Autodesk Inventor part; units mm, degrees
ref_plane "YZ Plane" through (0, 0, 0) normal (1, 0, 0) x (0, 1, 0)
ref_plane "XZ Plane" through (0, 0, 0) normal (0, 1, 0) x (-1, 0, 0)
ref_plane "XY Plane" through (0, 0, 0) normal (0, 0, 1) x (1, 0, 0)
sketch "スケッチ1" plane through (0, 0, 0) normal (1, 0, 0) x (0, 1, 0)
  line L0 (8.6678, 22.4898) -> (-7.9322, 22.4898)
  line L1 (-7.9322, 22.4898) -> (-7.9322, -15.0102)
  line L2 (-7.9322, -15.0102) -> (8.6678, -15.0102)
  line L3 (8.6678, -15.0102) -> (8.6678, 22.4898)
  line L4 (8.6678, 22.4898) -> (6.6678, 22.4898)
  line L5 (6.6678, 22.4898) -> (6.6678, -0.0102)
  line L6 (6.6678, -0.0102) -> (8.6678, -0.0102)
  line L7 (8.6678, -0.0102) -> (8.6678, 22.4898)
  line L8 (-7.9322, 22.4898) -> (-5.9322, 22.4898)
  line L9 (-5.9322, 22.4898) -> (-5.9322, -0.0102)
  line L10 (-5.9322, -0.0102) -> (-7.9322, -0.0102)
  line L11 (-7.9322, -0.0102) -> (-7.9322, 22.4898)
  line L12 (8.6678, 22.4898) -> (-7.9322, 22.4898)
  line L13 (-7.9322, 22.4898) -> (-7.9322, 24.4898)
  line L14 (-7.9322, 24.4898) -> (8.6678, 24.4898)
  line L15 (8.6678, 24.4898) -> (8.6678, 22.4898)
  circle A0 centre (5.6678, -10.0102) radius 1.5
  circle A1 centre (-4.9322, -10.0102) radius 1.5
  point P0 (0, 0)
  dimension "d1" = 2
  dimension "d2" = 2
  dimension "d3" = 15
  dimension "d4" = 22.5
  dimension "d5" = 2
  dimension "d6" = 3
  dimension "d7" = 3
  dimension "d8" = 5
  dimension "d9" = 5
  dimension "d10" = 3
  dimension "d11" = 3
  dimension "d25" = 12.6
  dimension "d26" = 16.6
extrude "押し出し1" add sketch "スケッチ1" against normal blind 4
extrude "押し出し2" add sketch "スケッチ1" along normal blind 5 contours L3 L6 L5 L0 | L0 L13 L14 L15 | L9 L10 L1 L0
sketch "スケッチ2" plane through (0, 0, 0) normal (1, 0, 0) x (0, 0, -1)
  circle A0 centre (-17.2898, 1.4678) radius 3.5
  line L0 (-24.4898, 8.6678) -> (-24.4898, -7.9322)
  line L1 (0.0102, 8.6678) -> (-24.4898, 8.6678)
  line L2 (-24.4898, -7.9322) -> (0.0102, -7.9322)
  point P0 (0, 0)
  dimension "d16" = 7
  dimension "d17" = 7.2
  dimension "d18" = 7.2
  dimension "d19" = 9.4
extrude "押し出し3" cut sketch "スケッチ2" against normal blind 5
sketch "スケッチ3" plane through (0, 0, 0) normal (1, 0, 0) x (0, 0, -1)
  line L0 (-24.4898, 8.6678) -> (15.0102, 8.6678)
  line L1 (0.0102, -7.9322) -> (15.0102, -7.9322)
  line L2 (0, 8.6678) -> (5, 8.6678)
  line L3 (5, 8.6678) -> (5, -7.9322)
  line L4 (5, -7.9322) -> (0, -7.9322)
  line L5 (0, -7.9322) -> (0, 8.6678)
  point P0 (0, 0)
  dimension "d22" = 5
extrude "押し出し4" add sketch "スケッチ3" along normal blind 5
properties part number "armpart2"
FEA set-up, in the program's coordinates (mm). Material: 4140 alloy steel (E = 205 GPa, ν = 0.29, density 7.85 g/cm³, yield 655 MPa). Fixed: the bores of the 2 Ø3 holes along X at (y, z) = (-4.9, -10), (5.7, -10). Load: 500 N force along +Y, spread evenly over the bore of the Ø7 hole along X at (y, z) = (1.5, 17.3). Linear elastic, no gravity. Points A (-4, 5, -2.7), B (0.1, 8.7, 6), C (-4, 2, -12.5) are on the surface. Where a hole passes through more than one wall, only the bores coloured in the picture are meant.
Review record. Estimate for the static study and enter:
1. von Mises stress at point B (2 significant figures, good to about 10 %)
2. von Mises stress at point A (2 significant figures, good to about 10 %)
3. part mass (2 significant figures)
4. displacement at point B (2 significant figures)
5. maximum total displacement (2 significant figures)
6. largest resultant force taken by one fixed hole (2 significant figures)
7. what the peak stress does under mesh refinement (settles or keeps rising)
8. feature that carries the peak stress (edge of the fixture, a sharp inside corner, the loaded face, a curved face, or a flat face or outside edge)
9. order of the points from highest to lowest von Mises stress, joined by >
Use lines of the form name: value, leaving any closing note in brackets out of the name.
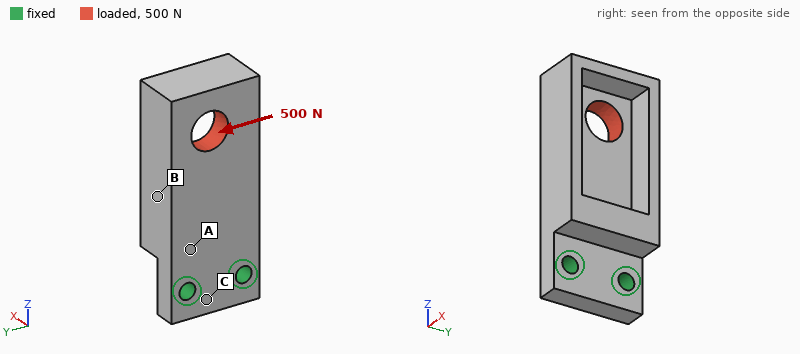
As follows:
von Mises stress at point B: 19 MPa
von Mises stress at point A: 37 MPa
part mass: 27 g
displacement at point B: 6.5 µm
maximum total displacement: 18 µm
largest resultant force taken by one fixed hole: 1.2 kN
what the peak stress does under mesh refinement: keeps rising
feature that carries the peak stress: edge of the fixture
order of the points from highest to lowest von Mises stress, joined by >: A > B > C
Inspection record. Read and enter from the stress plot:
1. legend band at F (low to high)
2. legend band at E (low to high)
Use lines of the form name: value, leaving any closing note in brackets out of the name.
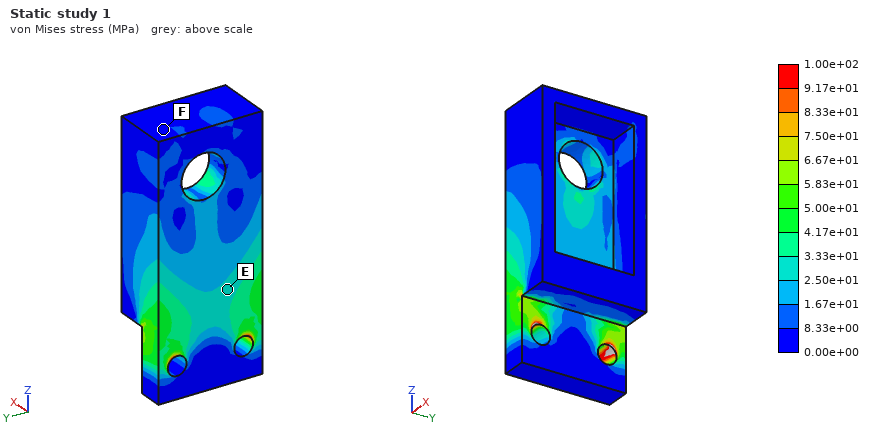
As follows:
legend band at F: 0.00e+00 to 8.33e+00 MPa
legend band at E: 2.50e+01 to 3.33e+01 MPa
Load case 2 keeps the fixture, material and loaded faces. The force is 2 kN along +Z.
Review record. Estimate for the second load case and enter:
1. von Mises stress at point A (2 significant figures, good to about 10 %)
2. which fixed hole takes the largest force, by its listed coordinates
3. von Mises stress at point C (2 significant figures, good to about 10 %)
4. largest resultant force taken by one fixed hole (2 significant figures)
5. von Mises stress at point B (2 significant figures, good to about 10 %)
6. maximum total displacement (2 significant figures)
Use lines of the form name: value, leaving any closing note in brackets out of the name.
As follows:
von Mises stress at point A: 44 MPa
which fixed hole takes the largest force, by its listed coordinates: (5.7, -10)
von Mises stress at point C: 10 MPa
largest resultant force taken by one fixed hole: 1.2 kN
von Mises stress at point B: 28 MPa
maximum total displacement: 12 µm
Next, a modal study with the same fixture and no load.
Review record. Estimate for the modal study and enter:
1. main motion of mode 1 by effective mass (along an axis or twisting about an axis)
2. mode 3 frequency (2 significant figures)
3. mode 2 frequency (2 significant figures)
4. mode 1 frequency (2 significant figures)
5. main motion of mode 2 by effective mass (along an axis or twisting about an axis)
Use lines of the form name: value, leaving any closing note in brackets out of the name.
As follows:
main motion of mode 1 by effective mass: along X
mode 3 frequency: 10 kHz
mode 2 frequency: 8200 Hz
mode 1 frequency: 3000 Hz
main motion of mode 2 by effective mass: along Y
